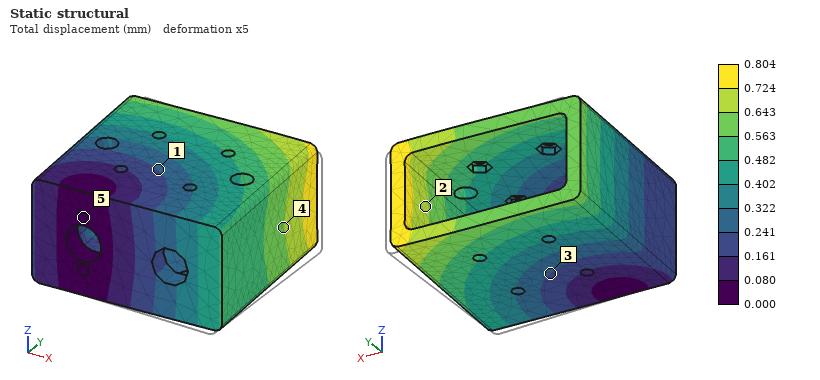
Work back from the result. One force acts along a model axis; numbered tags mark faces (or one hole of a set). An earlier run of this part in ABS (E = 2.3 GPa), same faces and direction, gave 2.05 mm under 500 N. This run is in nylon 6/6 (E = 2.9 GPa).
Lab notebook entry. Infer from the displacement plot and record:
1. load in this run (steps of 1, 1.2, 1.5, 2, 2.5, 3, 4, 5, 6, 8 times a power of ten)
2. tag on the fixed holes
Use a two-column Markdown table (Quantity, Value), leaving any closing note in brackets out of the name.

| Quantity | Value |
|---|---|
| load in this run | 250 N |
| tag on the fixed holes | 5 |
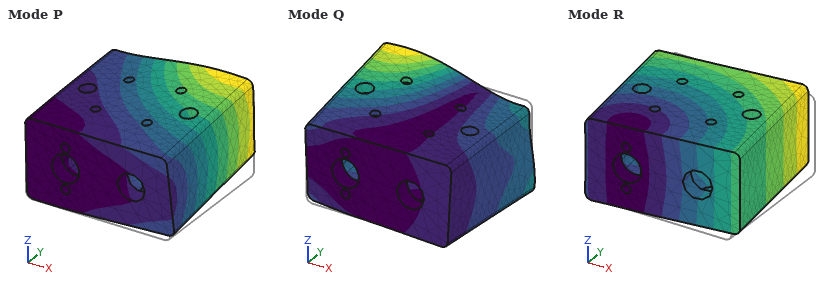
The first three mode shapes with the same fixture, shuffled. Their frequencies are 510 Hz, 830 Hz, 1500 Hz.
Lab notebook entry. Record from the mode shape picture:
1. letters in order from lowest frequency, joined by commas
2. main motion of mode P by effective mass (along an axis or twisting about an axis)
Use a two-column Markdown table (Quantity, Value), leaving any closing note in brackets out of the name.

| Quantity | Value |
|---|---|
| letters in order from lowest frequency, joined by commas | R, P, Q |
| main motion of mode P by effective mass | along Z |
